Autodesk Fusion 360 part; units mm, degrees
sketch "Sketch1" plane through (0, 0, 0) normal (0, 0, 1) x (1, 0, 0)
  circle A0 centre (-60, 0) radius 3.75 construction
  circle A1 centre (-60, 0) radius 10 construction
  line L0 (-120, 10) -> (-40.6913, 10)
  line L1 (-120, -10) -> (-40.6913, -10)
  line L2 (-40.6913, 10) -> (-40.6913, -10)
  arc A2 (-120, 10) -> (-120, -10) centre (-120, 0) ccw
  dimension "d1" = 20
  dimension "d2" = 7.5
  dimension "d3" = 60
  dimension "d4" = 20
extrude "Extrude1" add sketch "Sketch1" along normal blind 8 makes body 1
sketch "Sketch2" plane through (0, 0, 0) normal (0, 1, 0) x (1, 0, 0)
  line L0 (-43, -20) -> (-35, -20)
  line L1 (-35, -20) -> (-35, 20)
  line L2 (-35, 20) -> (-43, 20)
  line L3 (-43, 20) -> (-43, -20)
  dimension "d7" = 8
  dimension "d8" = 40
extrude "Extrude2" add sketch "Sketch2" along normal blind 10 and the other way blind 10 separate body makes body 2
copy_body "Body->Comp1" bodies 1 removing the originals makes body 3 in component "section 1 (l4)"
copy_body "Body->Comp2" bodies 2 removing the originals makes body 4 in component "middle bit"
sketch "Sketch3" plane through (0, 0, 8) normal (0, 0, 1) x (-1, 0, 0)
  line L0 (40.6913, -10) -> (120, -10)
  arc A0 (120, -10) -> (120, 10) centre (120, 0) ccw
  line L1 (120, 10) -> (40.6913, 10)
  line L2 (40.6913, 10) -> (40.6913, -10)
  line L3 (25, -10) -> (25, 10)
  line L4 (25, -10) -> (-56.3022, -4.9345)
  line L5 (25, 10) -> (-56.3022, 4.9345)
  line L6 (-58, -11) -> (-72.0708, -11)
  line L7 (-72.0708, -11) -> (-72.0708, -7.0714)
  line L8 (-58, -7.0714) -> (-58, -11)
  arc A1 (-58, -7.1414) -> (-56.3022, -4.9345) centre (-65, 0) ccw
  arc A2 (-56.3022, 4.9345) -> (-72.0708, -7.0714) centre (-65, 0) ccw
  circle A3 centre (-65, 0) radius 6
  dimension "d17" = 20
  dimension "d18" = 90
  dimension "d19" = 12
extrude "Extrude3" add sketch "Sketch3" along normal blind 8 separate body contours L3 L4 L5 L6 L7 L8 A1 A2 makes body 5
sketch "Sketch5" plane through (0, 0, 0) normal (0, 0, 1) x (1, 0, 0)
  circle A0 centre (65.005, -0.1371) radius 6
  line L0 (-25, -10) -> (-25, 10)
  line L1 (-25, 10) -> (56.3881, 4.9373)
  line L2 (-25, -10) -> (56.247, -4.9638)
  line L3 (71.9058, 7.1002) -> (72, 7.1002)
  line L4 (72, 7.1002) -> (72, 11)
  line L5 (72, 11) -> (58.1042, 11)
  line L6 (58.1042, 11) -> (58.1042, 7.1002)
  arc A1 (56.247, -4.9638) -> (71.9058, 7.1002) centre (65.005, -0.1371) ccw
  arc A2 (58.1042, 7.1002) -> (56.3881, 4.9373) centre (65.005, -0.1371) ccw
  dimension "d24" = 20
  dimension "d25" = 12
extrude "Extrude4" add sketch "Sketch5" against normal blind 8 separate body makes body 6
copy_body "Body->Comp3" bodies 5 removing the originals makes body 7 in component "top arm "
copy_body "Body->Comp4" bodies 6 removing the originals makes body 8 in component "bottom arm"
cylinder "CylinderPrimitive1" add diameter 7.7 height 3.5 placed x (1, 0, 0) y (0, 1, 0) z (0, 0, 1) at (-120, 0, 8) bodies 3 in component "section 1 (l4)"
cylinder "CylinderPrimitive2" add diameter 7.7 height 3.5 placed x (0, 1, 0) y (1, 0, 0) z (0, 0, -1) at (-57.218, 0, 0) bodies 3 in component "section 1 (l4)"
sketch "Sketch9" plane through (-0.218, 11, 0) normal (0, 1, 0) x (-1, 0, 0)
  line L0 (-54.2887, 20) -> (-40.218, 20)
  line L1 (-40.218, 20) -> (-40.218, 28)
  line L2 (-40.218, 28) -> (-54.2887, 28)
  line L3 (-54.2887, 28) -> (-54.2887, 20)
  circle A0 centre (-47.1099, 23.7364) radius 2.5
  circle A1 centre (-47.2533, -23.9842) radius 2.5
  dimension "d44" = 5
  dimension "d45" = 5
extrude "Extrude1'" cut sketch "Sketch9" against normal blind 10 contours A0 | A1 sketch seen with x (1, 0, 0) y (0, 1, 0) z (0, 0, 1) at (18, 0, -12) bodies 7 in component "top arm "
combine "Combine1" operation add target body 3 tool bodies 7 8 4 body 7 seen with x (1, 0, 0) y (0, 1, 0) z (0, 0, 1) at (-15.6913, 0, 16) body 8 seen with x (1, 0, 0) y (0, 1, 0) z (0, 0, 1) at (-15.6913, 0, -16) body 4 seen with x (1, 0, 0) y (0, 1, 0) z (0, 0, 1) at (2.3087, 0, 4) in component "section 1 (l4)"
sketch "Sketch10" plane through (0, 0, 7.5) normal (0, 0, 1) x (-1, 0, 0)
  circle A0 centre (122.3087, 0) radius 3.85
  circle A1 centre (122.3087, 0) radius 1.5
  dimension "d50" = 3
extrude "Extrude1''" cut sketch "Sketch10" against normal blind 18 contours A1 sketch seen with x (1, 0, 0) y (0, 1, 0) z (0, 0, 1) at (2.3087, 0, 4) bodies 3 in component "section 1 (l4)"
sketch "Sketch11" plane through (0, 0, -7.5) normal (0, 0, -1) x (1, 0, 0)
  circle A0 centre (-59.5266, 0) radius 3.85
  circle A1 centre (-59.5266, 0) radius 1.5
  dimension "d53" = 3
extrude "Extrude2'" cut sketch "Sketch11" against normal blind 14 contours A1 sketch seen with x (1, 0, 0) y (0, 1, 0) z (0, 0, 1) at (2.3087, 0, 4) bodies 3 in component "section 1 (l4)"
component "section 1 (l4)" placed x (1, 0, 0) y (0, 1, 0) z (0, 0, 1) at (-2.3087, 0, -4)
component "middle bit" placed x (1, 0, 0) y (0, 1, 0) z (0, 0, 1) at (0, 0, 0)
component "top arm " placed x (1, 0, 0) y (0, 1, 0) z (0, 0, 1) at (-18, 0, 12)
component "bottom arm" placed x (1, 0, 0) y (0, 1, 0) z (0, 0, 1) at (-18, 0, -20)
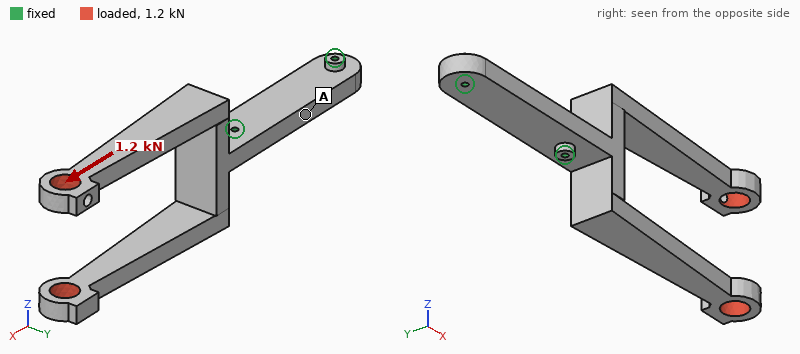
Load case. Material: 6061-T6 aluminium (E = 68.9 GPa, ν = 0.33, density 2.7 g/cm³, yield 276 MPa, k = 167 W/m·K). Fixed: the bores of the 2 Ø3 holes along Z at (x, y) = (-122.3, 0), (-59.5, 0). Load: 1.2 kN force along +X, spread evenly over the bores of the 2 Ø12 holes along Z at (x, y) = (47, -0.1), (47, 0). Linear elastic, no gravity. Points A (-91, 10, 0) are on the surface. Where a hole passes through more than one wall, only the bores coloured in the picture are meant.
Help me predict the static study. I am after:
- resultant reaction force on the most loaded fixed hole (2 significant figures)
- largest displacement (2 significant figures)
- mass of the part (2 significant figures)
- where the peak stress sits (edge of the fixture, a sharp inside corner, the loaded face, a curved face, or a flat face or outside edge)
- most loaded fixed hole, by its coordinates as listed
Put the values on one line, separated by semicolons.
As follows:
1.1 kN; 0.30 mm; 120 g; the loaded face; (-59.5, 0)
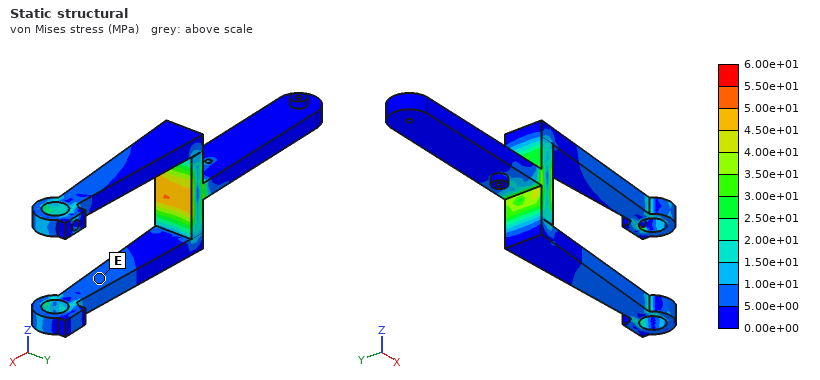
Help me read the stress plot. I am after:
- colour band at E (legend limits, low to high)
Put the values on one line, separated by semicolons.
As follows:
5.00e+00 to 1.00e+01 MPa
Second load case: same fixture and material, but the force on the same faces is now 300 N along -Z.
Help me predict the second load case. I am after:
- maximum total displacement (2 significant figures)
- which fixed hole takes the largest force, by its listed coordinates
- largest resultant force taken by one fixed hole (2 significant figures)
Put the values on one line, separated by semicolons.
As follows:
2.3 mm; (-59.5, 0); 390 N
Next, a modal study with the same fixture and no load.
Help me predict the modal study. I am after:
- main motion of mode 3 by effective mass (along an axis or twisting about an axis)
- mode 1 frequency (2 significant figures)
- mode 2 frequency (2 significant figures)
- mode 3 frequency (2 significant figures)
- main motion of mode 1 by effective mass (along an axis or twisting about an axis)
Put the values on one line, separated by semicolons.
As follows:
along Y; 420 Hz; 650 Hz; 730 Hz; along Z
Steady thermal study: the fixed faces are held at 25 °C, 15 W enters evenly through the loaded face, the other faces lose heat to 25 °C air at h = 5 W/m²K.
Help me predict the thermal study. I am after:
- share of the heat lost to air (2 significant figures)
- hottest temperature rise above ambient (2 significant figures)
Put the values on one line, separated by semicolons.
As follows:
10 %; 52 K
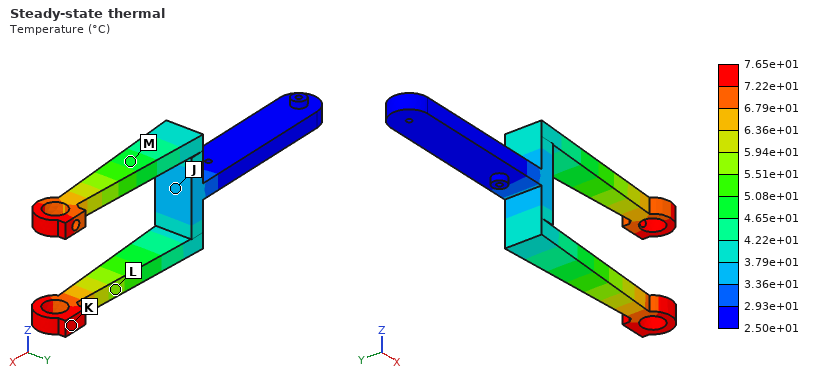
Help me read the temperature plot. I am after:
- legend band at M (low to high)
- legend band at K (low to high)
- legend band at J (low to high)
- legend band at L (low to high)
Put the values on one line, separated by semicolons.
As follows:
4.65e+01 to 5.08e+01 °C; 7.22e+01 to 7.65e+01 °C; 3.36e+01 to 3.79e+01 °C; 5.51e+01 to 5.94e+01 °C
